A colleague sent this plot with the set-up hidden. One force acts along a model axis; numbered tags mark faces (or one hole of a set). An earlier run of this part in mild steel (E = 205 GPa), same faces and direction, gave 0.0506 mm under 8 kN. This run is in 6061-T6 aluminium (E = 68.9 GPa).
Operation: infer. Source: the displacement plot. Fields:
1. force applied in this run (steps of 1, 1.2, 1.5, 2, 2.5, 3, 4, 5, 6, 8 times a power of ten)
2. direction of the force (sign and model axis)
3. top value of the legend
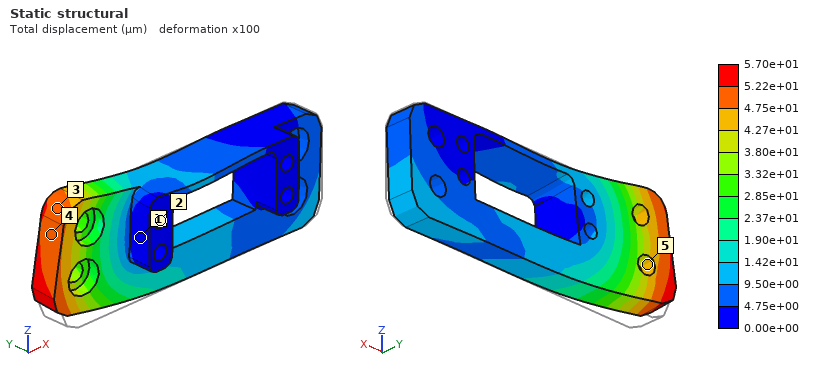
3 kN
+Z
5.70e+01 µm
